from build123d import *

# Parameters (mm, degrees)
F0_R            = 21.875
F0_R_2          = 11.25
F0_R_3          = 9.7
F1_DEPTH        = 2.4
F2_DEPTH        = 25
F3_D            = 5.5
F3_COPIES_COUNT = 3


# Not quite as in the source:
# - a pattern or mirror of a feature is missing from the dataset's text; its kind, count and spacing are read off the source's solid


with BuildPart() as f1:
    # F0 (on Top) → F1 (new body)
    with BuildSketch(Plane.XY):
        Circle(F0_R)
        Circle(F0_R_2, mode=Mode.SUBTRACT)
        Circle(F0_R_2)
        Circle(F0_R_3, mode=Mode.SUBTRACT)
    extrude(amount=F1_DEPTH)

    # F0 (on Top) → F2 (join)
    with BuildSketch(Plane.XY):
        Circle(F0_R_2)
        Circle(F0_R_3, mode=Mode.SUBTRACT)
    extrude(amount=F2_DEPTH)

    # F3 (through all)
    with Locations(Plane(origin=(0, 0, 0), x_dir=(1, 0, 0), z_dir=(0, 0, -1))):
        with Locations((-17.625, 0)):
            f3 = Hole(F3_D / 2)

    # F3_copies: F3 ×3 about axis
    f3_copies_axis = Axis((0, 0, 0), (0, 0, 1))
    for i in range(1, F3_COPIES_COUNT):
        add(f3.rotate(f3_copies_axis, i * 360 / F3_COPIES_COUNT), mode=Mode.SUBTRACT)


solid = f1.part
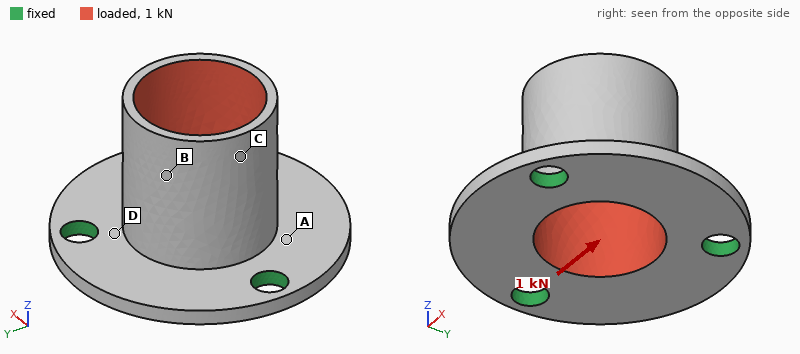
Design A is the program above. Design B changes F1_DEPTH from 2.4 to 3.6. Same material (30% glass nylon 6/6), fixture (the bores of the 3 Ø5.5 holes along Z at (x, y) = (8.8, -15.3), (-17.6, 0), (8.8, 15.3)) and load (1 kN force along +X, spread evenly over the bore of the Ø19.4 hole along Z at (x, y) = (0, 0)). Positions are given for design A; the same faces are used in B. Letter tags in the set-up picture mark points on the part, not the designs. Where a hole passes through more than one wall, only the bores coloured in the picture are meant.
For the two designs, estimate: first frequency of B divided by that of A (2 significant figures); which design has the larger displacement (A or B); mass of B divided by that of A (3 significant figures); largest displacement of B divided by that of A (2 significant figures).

1.3
A
1.25
0.55
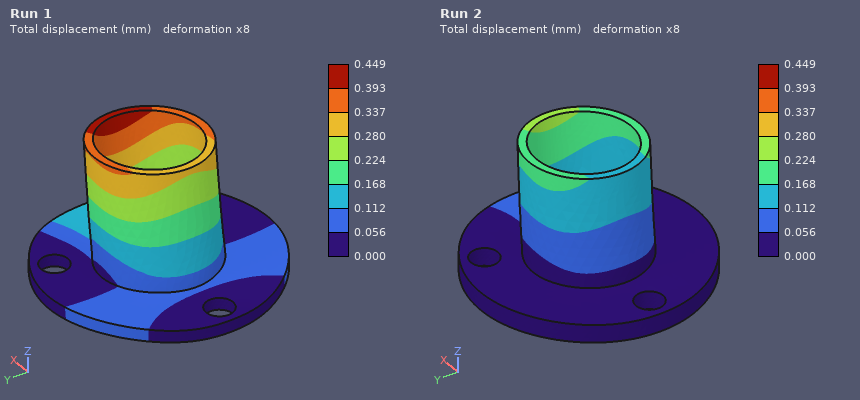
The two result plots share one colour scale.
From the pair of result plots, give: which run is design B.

Run 2
